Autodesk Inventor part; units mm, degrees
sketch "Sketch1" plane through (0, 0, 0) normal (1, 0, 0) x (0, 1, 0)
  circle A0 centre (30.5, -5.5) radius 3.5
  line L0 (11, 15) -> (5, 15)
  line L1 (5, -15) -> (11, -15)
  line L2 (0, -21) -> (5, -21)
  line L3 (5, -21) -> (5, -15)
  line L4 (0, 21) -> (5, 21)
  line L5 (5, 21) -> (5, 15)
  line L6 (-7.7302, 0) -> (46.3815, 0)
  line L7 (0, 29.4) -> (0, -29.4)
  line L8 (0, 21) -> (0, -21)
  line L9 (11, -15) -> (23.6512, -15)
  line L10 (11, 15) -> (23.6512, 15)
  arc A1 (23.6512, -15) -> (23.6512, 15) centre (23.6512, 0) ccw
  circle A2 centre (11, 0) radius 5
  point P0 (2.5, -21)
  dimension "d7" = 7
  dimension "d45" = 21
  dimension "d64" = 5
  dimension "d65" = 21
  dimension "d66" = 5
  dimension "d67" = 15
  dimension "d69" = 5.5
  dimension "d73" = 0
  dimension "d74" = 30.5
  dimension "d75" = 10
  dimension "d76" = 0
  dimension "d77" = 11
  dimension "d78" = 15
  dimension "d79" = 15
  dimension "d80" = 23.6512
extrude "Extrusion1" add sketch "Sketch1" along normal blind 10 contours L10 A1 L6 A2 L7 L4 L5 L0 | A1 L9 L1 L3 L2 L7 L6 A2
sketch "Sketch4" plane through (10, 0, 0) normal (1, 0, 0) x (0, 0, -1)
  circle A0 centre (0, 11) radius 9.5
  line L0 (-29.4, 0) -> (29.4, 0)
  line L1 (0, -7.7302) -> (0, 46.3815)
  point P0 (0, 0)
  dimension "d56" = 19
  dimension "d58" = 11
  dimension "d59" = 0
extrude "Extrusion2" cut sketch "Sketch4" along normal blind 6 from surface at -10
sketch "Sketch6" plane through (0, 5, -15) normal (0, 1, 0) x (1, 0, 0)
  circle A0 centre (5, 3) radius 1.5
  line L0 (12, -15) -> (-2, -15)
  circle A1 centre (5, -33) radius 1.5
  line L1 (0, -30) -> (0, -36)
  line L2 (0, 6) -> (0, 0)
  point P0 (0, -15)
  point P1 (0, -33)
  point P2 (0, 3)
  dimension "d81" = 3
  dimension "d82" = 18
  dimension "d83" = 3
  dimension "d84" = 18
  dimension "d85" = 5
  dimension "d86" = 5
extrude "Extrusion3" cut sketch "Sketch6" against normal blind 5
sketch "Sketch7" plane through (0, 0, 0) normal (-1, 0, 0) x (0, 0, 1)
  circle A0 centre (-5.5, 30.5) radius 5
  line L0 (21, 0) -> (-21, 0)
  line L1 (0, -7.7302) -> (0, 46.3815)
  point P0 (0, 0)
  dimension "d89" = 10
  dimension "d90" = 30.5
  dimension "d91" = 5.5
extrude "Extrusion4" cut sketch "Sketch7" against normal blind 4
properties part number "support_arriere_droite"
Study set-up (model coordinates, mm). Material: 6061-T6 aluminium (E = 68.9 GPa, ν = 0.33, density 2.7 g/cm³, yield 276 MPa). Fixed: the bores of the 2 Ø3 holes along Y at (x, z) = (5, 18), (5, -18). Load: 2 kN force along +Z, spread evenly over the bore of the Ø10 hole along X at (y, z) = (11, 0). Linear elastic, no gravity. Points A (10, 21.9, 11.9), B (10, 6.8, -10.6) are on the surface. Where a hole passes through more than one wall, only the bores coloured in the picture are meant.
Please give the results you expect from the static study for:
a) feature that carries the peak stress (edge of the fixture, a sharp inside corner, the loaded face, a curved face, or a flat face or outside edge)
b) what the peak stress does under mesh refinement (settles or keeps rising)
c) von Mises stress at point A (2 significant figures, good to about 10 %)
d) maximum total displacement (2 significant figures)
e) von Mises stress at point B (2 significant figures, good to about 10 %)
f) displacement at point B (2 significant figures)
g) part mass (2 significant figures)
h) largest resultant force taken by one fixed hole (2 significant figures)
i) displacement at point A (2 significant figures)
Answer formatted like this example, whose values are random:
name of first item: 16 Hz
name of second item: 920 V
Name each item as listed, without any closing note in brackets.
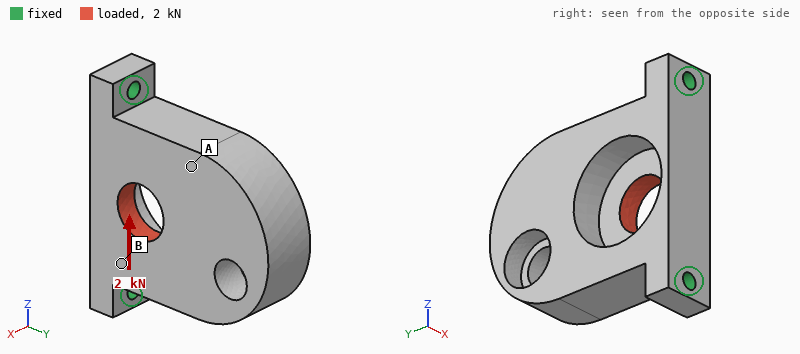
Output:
feature that carries the peak stress: a sharp inside corner
what the peak stress does under mesh refinement: keeps rising
von Mises stress at point A: 6.2 MPa
maximum total displacement: 13 µm
von Mises stress at point B: 28 MPa
displacement at point B: 4.9 µm
part mass: 23 g
largest resultant force taken by one fixed hole: 1.1 kN
displacement at point A: 12 µm
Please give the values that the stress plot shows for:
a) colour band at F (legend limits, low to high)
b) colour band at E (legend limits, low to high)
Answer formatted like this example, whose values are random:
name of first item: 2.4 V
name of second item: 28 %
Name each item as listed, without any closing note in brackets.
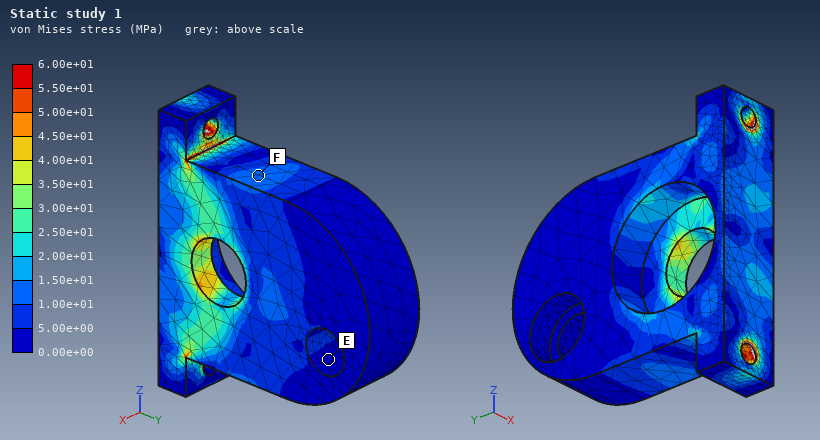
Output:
colour band at F: 1.00e+01 to 1.50e+01 MPa
colour band at E: 0.00e+00 to 5.00e+00 MPa
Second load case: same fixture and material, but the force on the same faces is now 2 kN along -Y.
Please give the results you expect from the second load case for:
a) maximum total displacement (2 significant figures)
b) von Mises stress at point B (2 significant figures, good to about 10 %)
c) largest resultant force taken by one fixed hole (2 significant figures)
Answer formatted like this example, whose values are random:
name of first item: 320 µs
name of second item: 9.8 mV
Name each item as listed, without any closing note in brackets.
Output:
maximum total displacement: 80 µm
von Mises stress at point B: 23 MPa
largest resultant force taken by one fixed hole: 1.1 kN
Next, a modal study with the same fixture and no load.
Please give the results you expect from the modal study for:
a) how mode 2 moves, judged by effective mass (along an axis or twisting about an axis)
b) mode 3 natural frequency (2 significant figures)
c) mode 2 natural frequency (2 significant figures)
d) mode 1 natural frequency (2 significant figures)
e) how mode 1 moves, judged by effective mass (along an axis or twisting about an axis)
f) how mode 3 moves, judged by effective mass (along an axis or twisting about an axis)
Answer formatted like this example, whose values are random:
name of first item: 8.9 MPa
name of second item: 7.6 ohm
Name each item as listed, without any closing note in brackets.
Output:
how mode 2 moves, judged by effective mass: along Z
mode 3 natural frequency: 12 kHz
mode 2 natural frequency: 9600 Hz
mode 1 natural frequency: 2900 Hz
how mode 1 moves, judged by effective mass: along X
how mode 3 moves, judged by effective mass: along Z
